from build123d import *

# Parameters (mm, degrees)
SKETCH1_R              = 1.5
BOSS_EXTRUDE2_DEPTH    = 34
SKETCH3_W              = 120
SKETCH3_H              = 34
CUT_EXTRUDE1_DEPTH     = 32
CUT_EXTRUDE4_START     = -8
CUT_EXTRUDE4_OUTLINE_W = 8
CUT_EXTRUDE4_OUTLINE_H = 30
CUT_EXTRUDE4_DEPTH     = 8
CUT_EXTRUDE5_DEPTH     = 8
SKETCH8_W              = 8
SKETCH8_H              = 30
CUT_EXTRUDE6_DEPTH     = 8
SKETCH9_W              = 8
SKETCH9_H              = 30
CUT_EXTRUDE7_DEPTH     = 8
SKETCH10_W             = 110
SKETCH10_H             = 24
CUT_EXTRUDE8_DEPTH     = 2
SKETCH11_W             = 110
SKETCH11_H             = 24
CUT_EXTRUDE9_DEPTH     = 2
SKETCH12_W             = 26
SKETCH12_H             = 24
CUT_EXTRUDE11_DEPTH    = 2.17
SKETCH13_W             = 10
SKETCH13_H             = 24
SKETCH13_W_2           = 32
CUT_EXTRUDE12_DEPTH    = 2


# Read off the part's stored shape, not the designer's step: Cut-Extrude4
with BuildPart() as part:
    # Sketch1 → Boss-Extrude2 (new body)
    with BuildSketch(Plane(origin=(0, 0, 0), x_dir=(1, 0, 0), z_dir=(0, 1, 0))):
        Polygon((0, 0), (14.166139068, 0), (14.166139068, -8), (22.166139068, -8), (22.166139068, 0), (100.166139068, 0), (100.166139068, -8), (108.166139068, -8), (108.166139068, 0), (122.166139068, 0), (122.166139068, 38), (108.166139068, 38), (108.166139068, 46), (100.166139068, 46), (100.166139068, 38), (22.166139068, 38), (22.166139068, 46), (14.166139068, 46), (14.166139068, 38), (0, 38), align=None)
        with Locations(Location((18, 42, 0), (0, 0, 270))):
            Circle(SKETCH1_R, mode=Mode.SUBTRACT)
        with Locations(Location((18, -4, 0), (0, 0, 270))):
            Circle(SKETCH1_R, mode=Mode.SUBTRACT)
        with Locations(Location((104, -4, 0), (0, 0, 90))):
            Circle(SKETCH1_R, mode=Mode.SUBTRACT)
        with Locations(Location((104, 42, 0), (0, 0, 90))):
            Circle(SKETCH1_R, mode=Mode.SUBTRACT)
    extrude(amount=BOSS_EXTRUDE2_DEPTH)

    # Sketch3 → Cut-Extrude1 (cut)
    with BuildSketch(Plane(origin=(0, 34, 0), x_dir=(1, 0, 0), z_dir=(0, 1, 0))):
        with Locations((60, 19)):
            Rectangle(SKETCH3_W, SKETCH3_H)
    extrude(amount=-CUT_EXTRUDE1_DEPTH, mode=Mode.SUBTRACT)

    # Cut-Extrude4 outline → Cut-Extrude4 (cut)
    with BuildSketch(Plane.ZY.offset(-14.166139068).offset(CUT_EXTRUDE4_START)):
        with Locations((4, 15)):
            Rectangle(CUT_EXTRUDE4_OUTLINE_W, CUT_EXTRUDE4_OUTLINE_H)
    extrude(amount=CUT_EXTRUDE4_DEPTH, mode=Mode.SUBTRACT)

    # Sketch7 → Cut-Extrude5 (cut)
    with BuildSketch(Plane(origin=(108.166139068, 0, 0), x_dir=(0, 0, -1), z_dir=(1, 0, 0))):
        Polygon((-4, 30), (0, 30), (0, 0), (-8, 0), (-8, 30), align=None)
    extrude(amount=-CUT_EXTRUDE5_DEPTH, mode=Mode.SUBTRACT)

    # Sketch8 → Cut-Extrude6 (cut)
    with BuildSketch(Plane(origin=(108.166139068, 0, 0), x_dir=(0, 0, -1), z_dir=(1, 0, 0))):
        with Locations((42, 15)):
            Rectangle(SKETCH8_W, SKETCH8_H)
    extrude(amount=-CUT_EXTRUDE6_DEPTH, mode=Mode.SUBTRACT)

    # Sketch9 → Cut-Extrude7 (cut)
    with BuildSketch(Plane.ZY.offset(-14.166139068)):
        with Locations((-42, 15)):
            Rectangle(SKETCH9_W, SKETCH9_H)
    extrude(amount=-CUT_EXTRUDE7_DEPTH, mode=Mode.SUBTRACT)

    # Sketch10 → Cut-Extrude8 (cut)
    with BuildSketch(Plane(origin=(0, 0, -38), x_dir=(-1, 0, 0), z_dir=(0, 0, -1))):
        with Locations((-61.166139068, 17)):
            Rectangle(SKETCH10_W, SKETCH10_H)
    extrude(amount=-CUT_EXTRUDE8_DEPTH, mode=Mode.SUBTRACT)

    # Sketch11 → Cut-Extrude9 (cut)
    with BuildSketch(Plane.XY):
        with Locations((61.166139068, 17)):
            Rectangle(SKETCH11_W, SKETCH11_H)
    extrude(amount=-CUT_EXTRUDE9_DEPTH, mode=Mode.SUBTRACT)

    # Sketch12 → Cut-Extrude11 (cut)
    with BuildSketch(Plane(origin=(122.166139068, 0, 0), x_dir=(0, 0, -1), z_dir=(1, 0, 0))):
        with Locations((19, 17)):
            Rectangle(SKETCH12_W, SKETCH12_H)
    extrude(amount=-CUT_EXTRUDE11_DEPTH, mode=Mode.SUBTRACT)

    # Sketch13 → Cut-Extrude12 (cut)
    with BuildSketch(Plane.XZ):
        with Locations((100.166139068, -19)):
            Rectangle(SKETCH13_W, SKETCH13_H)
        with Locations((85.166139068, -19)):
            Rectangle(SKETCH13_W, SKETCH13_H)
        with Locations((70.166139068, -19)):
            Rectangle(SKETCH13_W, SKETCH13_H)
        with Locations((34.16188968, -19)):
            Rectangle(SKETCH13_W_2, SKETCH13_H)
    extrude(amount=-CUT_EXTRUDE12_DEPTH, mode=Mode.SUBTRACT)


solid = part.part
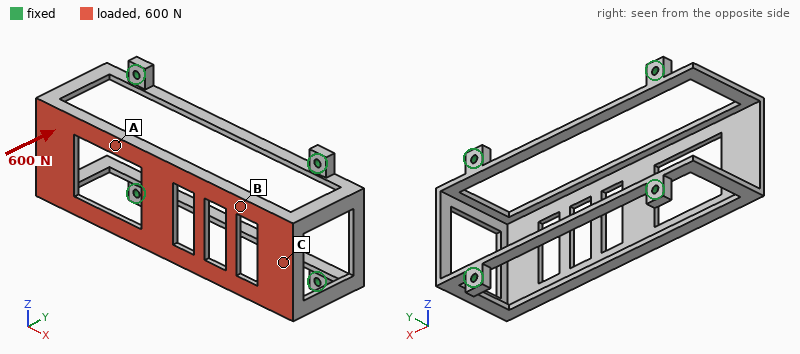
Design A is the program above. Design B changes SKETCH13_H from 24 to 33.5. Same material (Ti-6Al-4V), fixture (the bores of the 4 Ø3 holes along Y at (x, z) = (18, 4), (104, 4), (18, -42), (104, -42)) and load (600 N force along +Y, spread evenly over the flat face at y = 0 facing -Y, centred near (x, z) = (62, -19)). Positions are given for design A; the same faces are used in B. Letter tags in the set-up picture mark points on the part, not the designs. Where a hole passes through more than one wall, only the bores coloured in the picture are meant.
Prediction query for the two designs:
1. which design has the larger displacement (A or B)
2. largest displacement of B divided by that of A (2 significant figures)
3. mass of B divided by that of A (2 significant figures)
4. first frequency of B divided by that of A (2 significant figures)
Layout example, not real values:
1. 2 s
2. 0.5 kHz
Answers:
1. B
2. 1.1
3. 0.91
4. 1.1
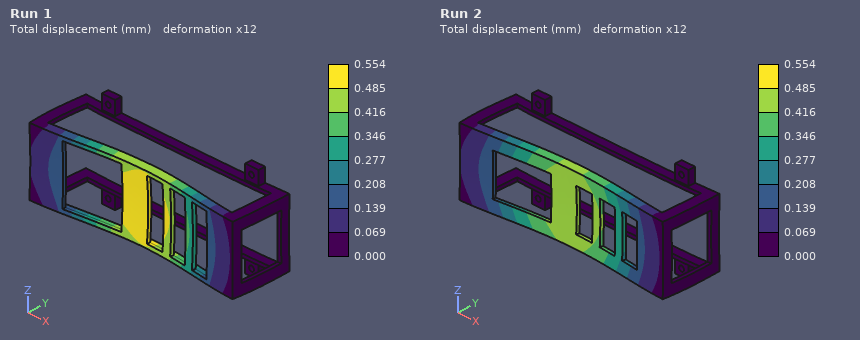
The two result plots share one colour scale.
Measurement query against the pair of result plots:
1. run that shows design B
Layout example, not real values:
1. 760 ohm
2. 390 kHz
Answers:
1. Run 1
